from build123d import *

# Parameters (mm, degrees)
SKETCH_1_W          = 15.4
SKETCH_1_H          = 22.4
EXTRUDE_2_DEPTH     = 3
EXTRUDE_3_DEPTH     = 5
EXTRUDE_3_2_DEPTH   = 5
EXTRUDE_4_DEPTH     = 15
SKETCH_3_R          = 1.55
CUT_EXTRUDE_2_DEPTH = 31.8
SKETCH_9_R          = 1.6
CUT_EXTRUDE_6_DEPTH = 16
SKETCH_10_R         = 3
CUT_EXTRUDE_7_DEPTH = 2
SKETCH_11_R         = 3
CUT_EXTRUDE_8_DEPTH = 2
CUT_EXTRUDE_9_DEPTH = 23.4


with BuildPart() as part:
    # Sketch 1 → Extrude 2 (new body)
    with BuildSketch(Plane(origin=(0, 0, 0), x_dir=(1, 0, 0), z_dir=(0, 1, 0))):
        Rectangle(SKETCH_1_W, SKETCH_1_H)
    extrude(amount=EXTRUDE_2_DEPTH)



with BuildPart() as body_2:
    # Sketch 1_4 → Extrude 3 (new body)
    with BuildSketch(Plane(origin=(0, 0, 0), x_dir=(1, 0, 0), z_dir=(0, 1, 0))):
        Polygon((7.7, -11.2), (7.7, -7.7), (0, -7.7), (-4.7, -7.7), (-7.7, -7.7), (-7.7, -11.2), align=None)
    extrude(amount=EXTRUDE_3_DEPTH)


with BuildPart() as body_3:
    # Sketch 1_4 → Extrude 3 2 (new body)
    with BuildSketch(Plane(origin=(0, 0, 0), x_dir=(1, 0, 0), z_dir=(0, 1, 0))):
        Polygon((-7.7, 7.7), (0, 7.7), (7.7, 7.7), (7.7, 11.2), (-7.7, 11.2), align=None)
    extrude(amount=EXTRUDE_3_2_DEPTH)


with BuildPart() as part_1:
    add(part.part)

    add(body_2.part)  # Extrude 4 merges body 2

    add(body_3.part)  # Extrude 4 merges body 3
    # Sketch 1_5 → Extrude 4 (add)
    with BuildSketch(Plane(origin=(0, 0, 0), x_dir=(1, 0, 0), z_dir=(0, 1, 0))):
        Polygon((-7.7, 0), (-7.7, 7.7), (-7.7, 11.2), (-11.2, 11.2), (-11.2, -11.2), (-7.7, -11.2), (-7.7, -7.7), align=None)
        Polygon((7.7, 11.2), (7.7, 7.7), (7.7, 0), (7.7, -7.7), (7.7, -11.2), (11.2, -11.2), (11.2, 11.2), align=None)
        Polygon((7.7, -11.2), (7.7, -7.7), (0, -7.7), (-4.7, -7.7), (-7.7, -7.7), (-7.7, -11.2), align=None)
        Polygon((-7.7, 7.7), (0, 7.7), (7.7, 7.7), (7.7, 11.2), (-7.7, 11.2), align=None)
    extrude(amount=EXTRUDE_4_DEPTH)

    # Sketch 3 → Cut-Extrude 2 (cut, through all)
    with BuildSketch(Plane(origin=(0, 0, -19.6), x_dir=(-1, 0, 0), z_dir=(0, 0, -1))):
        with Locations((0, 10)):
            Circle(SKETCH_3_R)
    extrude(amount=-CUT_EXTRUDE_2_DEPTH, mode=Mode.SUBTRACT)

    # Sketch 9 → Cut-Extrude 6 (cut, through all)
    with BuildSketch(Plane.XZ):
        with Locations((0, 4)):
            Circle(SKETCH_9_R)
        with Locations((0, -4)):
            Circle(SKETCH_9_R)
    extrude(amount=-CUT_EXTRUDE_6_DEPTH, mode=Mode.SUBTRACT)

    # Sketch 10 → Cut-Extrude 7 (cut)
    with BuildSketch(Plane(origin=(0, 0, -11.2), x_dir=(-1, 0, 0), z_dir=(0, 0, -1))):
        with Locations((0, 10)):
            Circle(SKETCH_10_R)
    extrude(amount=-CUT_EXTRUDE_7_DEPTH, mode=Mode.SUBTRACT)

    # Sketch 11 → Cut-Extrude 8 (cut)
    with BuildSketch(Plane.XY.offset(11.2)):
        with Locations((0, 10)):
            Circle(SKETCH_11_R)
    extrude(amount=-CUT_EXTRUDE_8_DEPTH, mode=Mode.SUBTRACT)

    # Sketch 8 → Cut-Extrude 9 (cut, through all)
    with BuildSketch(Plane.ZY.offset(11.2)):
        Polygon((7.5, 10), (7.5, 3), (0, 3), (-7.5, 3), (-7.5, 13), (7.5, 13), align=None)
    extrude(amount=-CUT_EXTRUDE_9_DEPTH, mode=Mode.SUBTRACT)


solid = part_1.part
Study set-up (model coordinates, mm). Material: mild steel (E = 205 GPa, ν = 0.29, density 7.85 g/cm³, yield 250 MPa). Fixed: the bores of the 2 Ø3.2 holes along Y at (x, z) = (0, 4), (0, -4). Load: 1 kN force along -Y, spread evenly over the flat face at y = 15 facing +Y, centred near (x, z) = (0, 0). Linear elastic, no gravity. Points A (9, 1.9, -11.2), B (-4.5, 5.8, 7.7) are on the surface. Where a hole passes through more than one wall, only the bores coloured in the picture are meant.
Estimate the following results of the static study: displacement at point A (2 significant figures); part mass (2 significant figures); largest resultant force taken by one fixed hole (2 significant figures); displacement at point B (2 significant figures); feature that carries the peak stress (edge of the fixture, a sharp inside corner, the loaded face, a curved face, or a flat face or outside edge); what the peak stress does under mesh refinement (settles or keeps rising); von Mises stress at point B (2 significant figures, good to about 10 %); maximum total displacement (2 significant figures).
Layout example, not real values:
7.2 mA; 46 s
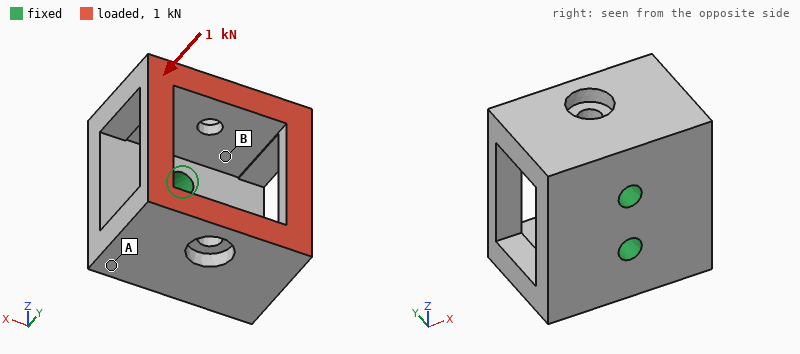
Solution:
3.3 µm; 27 g; 500 N; 2.6 µm; edge of the fixture; keeps rising; 28 MPa; 11 µm
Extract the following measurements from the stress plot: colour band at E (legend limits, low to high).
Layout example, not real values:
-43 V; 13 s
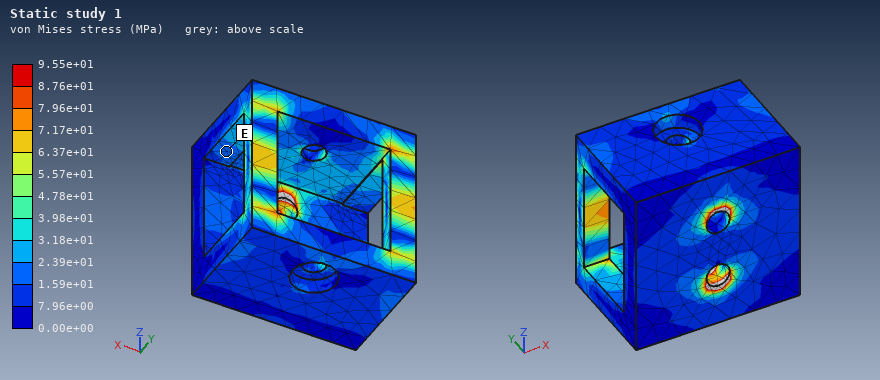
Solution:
1.59e+01 to 2.39e+01 MPa
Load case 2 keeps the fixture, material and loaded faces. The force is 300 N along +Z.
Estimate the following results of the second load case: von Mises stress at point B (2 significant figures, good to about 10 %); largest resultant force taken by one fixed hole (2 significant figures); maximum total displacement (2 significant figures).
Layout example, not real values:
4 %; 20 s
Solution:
17 MPa; 270 N; 16 µm
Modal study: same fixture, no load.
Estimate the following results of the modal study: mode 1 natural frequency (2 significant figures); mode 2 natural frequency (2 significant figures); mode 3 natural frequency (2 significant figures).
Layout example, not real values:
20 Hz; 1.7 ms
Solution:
8100 Hz; 8200 Hz; 12 kHz
